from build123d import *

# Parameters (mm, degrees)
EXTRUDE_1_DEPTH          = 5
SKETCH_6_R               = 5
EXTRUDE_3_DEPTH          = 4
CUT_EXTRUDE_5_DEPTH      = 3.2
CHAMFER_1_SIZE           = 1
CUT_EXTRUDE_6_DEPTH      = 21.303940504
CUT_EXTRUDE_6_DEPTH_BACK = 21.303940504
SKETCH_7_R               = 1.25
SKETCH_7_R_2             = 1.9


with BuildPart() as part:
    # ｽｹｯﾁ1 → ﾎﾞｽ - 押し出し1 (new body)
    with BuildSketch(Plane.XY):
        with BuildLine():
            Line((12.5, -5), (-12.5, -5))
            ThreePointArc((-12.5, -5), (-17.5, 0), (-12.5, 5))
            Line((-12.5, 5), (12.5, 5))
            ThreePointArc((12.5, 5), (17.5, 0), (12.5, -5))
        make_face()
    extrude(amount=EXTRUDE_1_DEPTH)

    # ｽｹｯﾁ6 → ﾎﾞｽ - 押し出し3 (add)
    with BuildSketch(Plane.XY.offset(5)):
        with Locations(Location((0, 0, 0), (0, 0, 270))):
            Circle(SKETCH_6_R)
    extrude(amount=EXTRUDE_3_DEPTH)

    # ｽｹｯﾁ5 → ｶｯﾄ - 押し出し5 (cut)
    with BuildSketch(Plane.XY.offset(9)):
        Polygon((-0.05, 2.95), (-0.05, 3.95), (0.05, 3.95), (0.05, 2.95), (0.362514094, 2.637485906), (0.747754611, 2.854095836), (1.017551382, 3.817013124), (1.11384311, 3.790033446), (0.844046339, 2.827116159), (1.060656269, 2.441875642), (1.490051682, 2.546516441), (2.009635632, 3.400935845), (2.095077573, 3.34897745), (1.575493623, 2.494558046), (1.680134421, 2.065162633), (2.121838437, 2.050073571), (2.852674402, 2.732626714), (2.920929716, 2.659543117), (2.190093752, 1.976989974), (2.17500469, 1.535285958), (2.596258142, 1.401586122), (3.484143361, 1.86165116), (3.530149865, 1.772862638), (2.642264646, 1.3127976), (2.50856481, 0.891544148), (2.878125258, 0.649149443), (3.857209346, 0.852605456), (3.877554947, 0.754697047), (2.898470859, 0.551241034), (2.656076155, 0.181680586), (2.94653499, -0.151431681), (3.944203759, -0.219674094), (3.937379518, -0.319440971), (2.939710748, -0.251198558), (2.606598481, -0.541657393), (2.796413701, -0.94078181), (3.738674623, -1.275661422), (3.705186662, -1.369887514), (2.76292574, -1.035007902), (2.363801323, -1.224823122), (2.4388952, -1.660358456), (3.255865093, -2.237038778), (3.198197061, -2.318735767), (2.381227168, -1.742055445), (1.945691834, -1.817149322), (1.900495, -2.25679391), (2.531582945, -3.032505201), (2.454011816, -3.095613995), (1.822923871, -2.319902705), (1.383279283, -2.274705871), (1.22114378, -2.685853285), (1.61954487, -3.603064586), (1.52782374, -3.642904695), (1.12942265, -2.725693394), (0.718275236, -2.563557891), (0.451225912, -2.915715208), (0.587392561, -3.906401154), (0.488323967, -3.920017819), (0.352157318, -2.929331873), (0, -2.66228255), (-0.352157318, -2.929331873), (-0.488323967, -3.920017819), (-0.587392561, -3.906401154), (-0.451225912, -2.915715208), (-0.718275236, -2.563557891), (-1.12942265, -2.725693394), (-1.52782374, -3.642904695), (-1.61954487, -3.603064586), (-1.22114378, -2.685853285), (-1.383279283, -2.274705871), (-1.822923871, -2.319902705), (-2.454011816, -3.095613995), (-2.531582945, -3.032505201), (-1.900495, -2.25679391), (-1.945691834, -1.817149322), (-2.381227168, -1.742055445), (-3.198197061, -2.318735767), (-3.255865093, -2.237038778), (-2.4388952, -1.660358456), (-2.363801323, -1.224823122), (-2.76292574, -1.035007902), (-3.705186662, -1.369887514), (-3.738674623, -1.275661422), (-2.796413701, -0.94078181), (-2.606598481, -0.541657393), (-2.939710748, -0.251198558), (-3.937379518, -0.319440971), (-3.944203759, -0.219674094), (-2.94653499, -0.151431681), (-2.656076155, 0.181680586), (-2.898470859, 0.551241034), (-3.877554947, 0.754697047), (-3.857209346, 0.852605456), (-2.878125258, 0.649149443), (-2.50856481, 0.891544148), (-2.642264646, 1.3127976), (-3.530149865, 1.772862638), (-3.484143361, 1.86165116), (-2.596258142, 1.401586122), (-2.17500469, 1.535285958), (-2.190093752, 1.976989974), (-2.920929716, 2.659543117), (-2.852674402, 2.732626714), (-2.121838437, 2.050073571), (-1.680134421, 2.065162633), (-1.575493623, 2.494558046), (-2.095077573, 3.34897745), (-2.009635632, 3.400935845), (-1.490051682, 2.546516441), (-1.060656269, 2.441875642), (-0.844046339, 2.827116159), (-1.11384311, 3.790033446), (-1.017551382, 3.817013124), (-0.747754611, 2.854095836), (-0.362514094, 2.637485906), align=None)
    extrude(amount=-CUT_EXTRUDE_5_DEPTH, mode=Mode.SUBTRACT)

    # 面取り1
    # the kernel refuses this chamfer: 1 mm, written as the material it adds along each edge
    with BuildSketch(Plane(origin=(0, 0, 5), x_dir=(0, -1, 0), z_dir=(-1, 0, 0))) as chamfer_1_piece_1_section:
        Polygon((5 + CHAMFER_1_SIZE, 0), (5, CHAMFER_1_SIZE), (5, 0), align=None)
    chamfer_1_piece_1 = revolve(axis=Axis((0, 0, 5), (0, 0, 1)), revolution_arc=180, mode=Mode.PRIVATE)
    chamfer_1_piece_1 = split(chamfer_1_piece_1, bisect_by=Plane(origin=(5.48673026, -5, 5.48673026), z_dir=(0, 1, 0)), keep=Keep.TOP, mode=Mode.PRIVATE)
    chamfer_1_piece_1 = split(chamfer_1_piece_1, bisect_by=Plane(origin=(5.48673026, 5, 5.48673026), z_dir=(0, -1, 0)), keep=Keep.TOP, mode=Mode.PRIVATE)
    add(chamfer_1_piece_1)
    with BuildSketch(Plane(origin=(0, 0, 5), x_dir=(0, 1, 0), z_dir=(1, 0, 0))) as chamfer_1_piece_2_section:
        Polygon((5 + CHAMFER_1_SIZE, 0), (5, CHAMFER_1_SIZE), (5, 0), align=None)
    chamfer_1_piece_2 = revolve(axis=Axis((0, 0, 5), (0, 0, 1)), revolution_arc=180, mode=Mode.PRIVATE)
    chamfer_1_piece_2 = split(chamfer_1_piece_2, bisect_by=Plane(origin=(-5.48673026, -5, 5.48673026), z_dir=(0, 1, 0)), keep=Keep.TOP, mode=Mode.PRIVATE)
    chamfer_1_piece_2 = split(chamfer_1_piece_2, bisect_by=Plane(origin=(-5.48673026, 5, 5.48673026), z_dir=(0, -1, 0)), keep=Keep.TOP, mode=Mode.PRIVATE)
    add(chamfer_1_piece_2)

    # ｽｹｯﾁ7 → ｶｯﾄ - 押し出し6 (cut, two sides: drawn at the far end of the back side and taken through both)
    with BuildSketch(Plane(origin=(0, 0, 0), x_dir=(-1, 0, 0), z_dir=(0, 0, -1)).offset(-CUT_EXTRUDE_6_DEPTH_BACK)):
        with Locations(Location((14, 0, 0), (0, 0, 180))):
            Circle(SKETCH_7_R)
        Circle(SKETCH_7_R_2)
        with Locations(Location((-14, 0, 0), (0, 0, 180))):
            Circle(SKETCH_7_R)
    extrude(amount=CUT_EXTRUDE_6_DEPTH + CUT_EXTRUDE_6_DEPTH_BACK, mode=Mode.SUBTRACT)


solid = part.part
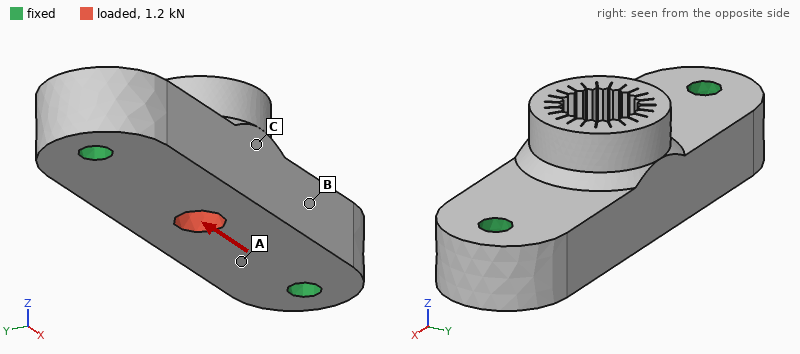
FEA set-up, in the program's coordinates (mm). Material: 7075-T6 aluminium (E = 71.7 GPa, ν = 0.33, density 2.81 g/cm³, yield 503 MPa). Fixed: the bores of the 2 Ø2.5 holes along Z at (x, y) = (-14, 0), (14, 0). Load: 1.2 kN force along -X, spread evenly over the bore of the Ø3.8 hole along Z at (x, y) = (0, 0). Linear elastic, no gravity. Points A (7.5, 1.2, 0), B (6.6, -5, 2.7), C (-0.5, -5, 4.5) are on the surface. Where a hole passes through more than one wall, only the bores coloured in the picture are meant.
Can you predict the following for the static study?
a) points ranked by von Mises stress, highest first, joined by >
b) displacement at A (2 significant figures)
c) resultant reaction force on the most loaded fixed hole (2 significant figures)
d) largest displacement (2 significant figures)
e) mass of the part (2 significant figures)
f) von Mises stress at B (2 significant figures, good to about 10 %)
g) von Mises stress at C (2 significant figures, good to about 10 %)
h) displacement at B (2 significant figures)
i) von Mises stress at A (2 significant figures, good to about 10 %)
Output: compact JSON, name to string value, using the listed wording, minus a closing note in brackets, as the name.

{"points ranked by von Mises stress, highest first, joined by >": "A > B > C", "displacement at A": "1.4 µm", "resultant reaction force on the most loaded fixed hole": "600 N", "largest displacement": "2.8 µm", "mass of the part": "5.0 g", "von Mises stress at B": "9.2 MPa", "von Mises stress at C": "3.1 MPa", "displacement at B": "1.6 µm", "von Mises stress at A": "13 MPa"}
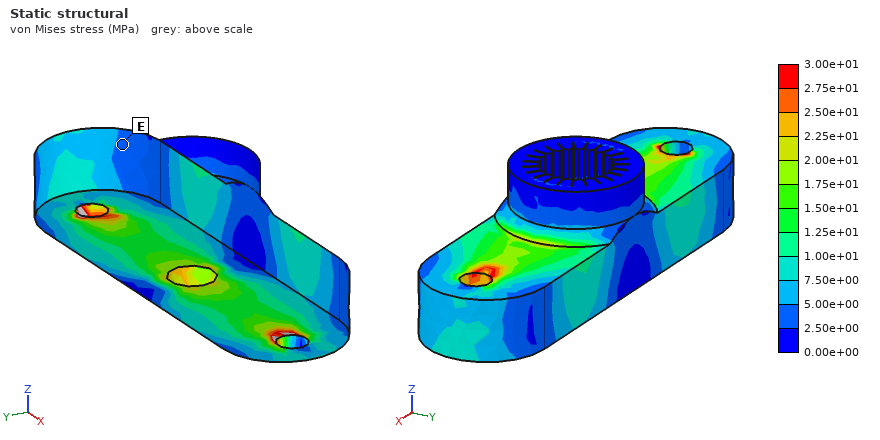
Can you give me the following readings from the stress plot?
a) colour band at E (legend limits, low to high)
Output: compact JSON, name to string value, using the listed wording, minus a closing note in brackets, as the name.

{"colour band at E": "2.50e+00 to 5.00e+00 MPa"}
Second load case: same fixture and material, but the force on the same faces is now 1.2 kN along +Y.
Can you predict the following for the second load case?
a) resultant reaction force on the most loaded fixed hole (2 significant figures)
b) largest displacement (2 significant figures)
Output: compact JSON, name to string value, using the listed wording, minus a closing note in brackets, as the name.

{"resultant reaction force on the most loaded fixed hole": "600 N", "largest displacement": "16 µm"}
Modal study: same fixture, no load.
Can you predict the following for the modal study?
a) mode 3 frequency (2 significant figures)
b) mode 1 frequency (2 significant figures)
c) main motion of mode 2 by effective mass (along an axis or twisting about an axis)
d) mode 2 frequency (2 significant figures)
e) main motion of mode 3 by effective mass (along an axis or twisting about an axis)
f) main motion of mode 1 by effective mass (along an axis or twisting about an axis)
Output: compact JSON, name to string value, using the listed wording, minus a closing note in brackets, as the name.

{"mode 3 frequency": "36 kHz", "mode 1 frequency": "26 kHz", "main motion of mode 2 by effective mass": "along Y", "mode 2 frequency": "27 kHz", "main motion of mode 3 by effective mass": "along Y", "main motion of mode 1 by effective mass": "along Z"}
